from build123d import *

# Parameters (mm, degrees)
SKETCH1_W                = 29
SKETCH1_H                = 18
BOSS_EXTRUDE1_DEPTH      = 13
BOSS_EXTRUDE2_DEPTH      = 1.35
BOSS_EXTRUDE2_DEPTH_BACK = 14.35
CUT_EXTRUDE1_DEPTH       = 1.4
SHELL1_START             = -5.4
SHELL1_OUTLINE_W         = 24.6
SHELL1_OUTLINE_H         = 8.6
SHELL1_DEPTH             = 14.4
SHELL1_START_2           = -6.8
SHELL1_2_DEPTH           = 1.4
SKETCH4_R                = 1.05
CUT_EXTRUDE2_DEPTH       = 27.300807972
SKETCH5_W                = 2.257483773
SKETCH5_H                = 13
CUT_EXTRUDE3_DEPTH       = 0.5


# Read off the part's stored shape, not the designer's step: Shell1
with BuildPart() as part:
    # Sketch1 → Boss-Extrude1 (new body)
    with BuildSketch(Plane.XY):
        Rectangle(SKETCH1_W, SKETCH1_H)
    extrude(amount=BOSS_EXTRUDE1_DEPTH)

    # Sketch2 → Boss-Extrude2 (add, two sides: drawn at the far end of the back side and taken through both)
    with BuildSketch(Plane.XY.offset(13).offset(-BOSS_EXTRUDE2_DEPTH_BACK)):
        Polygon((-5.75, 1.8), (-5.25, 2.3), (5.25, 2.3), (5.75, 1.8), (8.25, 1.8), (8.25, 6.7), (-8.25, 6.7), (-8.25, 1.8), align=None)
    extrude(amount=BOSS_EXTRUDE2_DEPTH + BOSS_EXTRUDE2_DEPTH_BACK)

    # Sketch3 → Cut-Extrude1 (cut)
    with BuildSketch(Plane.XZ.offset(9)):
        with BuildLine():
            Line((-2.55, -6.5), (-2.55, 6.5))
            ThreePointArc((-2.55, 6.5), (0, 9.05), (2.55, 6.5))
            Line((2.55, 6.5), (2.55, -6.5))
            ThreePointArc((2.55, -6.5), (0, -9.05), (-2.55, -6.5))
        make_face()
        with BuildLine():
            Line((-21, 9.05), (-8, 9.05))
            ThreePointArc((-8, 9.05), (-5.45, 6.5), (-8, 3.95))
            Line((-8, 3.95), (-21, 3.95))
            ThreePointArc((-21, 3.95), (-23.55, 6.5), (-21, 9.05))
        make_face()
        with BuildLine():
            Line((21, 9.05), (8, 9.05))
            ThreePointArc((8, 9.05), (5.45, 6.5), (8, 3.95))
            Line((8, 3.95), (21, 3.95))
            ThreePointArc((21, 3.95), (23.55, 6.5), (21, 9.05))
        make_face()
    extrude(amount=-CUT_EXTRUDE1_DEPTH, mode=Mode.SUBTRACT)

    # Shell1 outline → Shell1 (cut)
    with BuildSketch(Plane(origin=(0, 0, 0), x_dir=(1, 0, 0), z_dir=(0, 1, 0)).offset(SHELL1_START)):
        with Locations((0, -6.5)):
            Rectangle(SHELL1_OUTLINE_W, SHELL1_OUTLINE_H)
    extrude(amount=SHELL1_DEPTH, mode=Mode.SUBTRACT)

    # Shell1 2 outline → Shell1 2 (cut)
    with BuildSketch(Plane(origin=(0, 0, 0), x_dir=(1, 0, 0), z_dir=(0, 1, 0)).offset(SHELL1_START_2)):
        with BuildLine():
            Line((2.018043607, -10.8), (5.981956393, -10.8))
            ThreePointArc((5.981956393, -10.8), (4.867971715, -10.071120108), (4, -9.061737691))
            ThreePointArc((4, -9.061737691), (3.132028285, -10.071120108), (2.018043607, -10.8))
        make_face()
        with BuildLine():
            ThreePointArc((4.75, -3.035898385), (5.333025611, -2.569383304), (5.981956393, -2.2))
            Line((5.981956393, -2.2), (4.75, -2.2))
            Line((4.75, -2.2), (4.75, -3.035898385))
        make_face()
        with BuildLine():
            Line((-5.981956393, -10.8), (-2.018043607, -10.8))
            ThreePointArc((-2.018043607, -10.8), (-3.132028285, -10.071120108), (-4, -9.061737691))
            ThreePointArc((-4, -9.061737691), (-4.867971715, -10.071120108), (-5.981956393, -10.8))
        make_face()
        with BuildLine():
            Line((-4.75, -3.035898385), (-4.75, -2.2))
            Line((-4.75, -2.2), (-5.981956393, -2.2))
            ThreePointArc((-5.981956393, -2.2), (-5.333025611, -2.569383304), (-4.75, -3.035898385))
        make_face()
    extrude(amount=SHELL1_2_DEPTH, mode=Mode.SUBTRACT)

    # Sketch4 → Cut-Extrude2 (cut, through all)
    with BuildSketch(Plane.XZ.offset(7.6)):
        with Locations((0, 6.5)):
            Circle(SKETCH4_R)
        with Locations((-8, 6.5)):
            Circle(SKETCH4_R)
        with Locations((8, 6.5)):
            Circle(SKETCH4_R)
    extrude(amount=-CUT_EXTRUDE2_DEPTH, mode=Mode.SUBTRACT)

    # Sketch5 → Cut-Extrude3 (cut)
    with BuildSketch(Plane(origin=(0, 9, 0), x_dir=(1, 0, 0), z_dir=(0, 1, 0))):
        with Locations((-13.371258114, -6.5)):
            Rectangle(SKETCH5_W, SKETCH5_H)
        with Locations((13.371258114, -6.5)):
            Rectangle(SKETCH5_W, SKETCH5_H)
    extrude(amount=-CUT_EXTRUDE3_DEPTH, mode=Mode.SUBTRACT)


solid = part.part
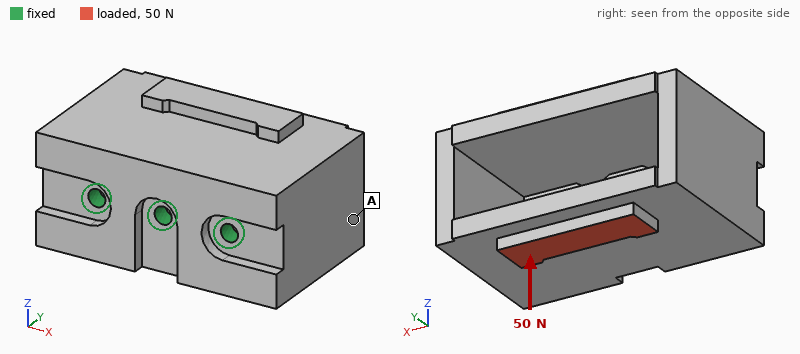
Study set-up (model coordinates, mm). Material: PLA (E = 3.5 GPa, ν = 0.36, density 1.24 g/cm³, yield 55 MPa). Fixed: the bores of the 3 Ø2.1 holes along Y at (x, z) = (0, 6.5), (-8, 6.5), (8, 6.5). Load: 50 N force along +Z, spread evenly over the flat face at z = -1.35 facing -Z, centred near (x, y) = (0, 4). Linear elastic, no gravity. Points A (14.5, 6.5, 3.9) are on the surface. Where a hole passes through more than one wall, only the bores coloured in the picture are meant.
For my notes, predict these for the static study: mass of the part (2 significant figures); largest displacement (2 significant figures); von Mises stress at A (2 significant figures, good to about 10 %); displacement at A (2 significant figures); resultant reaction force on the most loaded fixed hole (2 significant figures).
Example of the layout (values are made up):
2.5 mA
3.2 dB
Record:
4.6 g
0.23 mm
4.1 MPa
0.11 mm
27 N
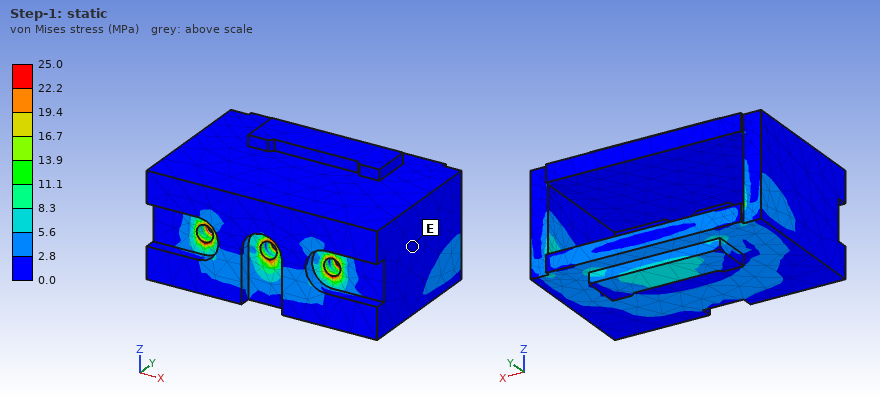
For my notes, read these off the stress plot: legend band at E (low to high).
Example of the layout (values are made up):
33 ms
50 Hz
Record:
0.0 to 2.8 MPa
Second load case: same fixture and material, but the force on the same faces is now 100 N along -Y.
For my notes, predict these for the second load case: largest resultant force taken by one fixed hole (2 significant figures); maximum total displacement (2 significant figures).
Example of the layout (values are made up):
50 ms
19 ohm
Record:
37 N
0.25 mm
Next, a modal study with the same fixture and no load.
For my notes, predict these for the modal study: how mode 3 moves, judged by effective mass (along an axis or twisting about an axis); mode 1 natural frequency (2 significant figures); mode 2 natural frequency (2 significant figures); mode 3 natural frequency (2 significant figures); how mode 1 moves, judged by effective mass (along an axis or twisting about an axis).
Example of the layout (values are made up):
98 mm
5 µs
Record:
along X
2100 Hz
4000 Hz
4600 Hz
along Z
